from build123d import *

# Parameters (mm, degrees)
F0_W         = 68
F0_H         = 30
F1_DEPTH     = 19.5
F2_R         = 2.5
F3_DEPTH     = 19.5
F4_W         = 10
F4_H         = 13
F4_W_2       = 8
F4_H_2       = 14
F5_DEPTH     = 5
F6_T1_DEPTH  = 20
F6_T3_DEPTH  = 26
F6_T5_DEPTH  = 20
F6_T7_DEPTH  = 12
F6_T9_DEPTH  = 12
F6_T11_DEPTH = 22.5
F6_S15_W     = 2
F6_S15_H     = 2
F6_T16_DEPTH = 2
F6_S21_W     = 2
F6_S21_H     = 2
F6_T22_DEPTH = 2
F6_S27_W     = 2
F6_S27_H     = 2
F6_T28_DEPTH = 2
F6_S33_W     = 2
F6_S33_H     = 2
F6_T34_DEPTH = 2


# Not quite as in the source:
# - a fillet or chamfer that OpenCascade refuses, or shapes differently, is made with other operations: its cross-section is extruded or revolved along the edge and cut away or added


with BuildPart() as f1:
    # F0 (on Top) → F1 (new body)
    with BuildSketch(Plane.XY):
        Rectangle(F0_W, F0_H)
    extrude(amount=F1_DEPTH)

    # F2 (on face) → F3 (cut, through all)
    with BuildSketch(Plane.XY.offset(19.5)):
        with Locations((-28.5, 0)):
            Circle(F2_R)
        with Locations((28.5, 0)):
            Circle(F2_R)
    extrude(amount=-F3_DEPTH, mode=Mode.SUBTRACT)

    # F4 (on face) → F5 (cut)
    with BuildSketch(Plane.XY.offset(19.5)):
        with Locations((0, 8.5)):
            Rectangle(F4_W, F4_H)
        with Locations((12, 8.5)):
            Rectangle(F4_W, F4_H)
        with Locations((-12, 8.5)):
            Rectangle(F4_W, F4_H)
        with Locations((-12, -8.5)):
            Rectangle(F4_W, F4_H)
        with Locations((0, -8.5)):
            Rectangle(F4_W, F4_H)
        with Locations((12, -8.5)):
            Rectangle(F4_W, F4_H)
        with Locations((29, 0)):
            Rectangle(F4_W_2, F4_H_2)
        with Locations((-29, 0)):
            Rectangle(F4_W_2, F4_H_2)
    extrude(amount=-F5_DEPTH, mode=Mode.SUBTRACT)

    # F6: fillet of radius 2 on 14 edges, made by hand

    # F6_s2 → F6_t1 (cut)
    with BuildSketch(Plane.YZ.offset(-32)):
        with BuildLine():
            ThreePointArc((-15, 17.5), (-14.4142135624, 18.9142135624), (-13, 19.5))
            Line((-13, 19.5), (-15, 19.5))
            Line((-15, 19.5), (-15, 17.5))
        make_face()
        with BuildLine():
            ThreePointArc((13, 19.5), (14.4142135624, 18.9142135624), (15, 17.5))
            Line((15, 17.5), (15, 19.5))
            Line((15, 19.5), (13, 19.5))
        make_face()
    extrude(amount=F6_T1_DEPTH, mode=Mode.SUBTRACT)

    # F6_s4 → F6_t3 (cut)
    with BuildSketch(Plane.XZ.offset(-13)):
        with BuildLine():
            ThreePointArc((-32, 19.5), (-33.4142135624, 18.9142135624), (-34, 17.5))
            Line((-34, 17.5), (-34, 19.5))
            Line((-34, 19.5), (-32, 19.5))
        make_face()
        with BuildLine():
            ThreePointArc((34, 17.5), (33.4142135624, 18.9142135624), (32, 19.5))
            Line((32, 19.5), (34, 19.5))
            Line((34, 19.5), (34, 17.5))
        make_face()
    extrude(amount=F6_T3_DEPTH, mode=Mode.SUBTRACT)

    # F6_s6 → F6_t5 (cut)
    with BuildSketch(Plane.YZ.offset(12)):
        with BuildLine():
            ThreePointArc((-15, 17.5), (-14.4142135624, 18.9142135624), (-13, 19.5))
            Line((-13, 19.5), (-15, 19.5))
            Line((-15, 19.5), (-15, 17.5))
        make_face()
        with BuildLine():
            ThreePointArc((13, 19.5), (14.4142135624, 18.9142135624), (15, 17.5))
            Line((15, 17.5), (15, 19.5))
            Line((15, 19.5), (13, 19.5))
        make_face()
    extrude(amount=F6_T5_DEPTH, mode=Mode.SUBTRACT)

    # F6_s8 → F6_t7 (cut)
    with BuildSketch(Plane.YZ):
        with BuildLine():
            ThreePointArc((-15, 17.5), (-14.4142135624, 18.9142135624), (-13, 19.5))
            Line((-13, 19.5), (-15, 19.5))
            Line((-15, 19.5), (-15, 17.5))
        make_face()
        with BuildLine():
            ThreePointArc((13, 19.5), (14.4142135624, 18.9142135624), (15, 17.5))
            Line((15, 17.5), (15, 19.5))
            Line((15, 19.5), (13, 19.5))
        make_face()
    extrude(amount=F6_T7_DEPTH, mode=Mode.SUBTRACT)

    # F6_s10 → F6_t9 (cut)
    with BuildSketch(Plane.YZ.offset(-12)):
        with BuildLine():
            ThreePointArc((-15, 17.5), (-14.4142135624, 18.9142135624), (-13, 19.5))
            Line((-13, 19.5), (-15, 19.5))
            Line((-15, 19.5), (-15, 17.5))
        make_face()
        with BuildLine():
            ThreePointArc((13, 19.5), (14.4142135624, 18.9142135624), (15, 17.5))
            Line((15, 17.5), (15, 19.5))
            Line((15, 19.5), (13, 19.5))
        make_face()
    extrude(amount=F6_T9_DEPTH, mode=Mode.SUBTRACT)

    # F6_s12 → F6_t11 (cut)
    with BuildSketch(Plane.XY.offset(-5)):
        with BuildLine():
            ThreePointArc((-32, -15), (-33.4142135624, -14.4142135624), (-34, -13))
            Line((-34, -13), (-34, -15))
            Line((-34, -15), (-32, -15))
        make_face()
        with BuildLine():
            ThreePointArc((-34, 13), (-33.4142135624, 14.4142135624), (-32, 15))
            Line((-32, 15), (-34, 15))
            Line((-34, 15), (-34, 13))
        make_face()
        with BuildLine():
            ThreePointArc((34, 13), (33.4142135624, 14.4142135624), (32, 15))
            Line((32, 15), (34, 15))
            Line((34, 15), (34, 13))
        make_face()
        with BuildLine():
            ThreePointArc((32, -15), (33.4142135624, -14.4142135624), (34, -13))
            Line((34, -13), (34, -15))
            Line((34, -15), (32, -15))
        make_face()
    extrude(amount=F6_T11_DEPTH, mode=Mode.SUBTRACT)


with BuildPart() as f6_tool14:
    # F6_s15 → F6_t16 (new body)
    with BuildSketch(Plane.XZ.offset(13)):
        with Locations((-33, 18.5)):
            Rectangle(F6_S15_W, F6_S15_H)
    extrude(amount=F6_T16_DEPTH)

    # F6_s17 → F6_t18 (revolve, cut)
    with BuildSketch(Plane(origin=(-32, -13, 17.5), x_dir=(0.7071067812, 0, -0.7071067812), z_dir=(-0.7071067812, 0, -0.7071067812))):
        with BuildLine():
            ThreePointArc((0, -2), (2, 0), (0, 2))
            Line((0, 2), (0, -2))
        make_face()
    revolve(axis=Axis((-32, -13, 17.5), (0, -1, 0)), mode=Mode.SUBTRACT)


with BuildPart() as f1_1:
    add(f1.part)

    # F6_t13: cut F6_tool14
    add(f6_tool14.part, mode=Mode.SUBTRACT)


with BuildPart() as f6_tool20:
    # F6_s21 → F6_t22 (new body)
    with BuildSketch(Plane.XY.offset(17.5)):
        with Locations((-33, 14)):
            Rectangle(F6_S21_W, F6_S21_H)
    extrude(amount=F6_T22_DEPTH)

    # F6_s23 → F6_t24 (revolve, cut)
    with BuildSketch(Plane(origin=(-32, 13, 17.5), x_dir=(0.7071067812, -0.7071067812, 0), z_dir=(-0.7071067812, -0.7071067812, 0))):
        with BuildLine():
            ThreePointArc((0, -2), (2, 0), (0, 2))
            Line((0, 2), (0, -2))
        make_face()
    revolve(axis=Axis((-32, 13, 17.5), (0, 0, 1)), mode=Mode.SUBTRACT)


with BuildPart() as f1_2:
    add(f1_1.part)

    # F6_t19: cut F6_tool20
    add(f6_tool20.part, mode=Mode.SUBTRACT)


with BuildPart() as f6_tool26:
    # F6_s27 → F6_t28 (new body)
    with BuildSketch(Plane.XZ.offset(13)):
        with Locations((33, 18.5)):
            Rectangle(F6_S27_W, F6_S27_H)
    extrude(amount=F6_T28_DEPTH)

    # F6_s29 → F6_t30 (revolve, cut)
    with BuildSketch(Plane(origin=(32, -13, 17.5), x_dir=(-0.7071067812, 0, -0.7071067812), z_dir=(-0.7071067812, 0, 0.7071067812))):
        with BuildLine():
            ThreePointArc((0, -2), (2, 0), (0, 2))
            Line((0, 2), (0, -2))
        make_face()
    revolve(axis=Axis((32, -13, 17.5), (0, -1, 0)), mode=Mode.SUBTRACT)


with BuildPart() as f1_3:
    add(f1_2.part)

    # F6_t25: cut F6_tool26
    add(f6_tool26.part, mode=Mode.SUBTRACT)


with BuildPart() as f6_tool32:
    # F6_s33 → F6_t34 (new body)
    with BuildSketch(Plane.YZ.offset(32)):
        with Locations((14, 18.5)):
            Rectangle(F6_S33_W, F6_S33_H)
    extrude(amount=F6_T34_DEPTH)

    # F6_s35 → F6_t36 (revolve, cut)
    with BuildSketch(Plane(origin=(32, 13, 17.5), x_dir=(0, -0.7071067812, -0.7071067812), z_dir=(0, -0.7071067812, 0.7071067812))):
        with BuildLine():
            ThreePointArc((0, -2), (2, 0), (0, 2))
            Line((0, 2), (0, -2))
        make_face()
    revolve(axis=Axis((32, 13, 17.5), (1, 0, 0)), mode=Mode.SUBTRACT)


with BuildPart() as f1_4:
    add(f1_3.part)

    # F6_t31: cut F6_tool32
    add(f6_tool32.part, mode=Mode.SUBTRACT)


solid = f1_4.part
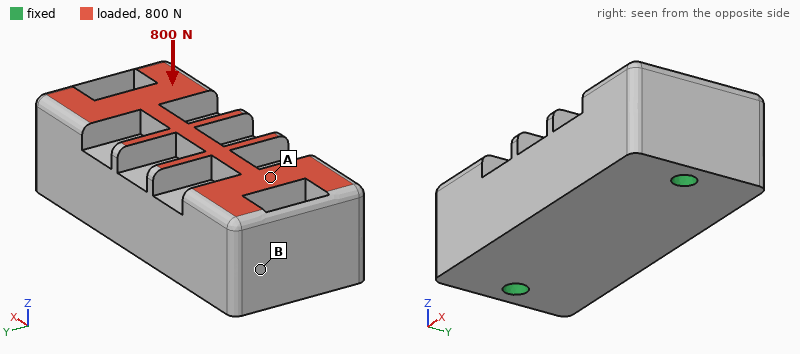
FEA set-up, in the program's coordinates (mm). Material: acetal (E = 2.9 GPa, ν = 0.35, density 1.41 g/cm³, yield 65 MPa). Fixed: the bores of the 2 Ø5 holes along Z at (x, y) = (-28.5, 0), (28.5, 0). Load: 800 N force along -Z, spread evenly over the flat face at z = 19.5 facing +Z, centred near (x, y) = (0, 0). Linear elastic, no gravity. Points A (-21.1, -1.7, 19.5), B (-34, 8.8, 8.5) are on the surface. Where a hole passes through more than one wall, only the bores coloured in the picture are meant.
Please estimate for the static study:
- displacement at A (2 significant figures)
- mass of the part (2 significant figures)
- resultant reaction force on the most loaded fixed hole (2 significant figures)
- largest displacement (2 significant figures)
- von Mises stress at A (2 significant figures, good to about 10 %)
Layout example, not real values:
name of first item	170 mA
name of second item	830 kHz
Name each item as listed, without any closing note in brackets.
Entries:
displacement at A	18 µm
mass of the part	48 g
resultant reaction force on the most loaded fixed hole	400 N
largest displacement	29 µm
von Mises stress at A	1.5 MPa
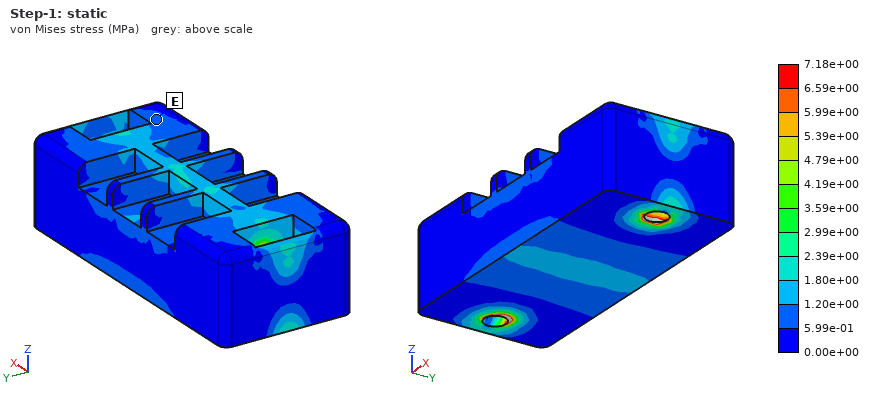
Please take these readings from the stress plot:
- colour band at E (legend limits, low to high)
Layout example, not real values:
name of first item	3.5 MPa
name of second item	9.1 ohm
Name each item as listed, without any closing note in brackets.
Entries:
colour band at E	5.99e-01 to 1.20e+00 MPa
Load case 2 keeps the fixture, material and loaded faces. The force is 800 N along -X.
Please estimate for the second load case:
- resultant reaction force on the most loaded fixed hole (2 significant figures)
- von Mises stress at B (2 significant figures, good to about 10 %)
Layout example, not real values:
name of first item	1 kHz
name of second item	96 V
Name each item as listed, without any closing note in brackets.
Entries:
resultant reaction force on the most loaded fixed hole	420 N
von Mises stress at B	1.2 MPa
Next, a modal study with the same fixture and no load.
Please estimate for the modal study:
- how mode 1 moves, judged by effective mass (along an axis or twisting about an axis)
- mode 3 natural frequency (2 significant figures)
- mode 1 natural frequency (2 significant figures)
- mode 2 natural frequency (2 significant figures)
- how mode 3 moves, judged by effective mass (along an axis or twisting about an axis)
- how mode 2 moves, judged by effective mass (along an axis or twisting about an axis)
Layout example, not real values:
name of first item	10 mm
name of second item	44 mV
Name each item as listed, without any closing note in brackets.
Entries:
how mode 1 moves, judged by effective mass	along Z
mode 3 natural frequency	4700 Hz
mode 1 natural frequency	4000 Hz
mode 2 natural frequency	4500 Hz
how mode 3 moves, judged by effective mass	along Y
how mode 2 moves, judged by effective mass	along Y
